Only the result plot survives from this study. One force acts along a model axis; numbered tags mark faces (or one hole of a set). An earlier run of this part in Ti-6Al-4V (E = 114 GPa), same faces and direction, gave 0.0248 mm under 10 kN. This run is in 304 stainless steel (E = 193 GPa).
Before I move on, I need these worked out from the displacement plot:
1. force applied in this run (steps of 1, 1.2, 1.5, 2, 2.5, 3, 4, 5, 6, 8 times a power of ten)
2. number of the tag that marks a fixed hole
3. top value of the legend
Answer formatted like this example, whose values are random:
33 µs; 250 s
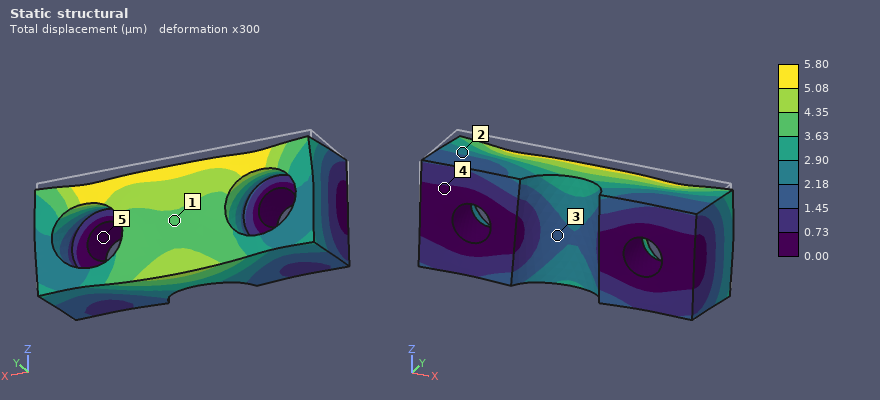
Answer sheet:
4 kN; 5; 5.80 µm
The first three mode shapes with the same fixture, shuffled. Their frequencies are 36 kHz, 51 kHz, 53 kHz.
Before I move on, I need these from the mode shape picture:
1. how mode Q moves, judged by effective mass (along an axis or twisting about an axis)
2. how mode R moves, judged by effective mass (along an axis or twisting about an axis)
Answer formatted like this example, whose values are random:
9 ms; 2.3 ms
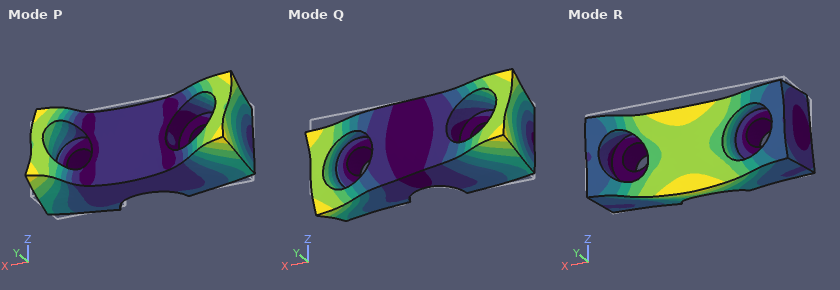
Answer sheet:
twisting about Y; along Z
